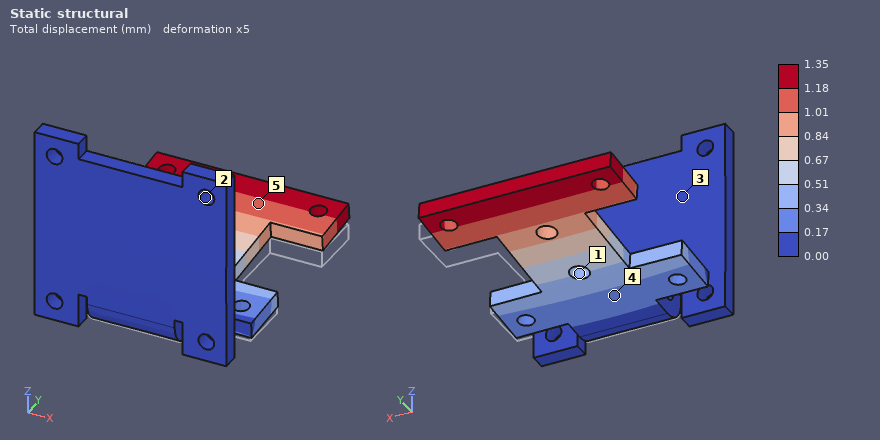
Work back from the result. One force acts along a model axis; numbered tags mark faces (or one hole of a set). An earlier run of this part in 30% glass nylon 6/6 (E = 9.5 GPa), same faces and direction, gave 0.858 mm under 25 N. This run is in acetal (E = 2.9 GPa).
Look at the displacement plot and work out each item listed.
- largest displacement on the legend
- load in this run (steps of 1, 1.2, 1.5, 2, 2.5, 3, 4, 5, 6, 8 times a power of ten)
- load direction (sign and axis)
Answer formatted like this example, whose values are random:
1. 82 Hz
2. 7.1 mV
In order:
1. 1.35 mm
2. 12 N
3. +Z
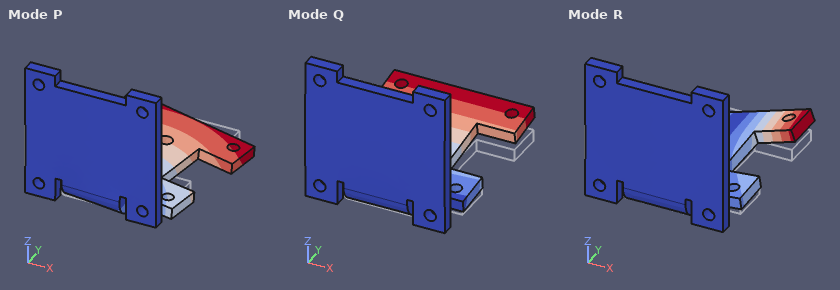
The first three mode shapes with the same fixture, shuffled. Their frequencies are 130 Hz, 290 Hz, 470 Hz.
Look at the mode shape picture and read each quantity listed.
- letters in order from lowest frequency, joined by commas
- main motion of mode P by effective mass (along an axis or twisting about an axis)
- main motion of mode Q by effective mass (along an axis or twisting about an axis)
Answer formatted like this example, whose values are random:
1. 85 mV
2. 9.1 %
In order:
1. Q, P, R
2. along X
3. along Z
